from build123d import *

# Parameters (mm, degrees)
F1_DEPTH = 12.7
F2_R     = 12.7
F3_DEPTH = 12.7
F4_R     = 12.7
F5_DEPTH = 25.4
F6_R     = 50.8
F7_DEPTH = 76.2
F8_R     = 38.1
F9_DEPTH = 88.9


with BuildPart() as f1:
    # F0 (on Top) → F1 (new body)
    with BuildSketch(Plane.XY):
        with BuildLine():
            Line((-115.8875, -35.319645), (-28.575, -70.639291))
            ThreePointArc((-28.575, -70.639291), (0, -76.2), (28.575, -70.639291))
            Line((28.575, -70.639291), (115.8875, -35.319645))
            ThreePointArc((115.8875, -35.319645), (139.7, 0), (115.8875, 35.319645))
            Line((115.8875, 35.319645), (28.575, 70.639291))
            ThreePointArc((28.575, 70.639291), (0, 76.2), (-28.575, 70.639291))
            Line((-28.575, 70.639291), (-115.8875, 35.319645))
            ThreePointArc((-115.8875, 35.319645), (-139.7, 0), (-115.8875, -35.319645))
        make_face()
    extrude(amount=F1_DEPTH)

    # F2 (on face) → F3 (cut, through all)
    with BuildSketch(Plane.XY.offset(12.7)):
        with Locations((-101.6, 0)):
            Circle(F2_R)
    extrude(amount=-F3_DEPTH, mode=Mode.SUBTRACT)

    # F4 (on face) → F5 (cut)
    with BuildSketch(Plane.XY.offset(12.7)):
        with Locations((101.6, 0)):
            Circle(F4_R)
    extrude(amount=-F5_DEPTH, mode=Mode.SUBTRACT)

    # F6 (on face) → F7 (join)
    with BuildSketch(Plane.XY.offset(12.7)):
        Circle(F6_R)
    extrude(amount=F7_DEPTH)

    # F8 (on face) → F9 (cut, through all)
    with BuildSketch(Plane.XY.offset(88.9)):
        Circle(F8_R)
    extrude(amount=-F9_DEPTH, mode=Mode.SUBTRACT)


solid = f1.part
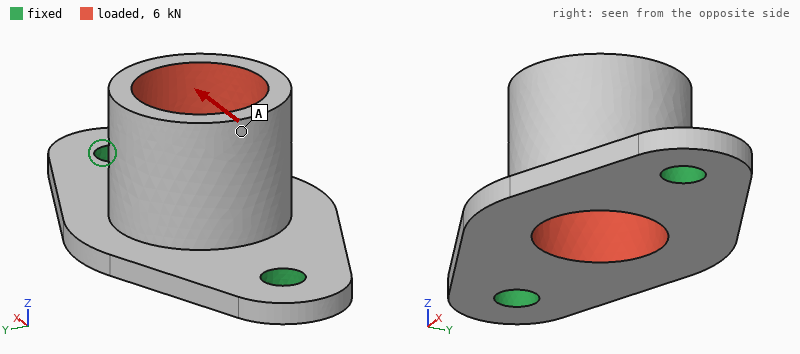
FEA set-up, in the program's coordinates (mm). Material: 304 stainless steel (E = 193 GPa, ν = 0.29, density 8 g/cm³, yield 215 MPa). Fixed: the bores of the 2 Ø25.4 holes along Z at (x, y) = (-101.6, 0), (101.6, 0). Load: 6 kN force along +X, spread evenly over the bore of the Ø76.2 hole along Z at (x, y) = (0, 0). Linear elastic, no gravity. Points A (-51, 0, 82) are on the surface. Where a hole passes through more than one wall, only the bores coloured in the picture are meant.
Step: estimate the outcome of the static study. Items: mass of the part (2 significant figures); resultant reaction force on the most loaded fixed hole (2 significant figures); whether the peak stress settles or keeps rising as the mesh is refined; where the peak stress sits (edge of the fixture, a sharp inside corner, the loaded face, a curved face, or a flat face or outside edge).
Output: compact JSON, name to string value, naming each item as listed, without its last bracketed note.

{"mass of the part": "4.6 kg", "resultant reaction force on the most loaded fixed hole": "3.4 kN", "whether the peak stress settles or keeps rising as the mesh is refined": "keeps rising", "where the peak stress sits": "edge of the fixture"}
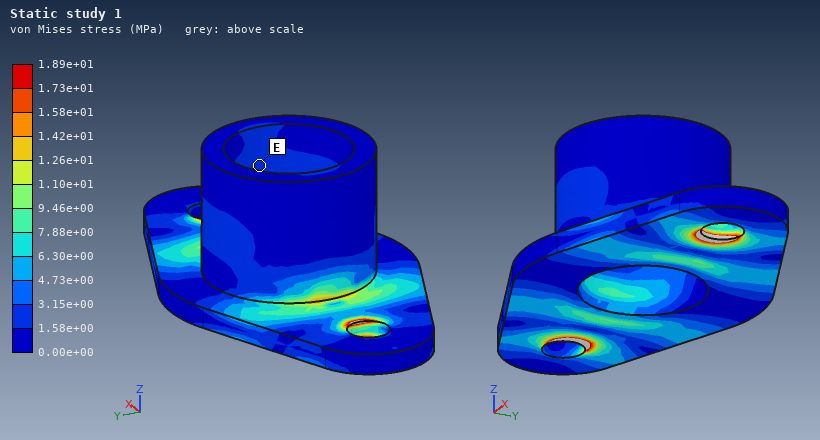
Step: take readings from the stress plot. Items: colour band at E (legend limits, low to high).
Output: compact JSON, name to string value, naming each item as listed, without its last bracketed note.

{"colour band at E": "1.58e+00 to 3.15e+00 MPa"}
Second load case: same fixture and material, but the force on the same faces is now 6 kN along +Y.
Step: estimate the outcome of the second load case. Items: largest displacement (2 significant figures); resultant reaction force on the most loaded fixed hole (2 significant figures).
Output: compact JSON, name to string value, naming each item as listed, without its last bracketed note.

{"largest displacement": "99 µm", "resultant reaction force on the most loaded fixed hole": "3.0 kN"}
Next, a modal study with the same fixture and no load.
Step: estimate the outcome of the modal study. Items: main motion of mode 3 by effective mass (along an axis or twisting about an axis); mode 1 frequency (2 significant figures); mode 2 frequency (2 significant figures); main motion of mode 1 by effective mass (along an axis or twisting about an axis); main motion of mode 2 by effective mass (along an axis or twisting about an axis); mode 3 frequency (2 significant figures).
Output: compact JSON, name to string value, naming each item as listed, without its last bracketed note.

{"main motion of mode 3 by effective mass": "along X", "mode 1 frequency": "760 Hz", "mode 2 frequency": "1500 Hz", "main motion of mode 1 by effective mass": "along Y", "main motion of mode 2 by effective mass": "along Z", "mode 3 frequency": "2100 Hz"}
